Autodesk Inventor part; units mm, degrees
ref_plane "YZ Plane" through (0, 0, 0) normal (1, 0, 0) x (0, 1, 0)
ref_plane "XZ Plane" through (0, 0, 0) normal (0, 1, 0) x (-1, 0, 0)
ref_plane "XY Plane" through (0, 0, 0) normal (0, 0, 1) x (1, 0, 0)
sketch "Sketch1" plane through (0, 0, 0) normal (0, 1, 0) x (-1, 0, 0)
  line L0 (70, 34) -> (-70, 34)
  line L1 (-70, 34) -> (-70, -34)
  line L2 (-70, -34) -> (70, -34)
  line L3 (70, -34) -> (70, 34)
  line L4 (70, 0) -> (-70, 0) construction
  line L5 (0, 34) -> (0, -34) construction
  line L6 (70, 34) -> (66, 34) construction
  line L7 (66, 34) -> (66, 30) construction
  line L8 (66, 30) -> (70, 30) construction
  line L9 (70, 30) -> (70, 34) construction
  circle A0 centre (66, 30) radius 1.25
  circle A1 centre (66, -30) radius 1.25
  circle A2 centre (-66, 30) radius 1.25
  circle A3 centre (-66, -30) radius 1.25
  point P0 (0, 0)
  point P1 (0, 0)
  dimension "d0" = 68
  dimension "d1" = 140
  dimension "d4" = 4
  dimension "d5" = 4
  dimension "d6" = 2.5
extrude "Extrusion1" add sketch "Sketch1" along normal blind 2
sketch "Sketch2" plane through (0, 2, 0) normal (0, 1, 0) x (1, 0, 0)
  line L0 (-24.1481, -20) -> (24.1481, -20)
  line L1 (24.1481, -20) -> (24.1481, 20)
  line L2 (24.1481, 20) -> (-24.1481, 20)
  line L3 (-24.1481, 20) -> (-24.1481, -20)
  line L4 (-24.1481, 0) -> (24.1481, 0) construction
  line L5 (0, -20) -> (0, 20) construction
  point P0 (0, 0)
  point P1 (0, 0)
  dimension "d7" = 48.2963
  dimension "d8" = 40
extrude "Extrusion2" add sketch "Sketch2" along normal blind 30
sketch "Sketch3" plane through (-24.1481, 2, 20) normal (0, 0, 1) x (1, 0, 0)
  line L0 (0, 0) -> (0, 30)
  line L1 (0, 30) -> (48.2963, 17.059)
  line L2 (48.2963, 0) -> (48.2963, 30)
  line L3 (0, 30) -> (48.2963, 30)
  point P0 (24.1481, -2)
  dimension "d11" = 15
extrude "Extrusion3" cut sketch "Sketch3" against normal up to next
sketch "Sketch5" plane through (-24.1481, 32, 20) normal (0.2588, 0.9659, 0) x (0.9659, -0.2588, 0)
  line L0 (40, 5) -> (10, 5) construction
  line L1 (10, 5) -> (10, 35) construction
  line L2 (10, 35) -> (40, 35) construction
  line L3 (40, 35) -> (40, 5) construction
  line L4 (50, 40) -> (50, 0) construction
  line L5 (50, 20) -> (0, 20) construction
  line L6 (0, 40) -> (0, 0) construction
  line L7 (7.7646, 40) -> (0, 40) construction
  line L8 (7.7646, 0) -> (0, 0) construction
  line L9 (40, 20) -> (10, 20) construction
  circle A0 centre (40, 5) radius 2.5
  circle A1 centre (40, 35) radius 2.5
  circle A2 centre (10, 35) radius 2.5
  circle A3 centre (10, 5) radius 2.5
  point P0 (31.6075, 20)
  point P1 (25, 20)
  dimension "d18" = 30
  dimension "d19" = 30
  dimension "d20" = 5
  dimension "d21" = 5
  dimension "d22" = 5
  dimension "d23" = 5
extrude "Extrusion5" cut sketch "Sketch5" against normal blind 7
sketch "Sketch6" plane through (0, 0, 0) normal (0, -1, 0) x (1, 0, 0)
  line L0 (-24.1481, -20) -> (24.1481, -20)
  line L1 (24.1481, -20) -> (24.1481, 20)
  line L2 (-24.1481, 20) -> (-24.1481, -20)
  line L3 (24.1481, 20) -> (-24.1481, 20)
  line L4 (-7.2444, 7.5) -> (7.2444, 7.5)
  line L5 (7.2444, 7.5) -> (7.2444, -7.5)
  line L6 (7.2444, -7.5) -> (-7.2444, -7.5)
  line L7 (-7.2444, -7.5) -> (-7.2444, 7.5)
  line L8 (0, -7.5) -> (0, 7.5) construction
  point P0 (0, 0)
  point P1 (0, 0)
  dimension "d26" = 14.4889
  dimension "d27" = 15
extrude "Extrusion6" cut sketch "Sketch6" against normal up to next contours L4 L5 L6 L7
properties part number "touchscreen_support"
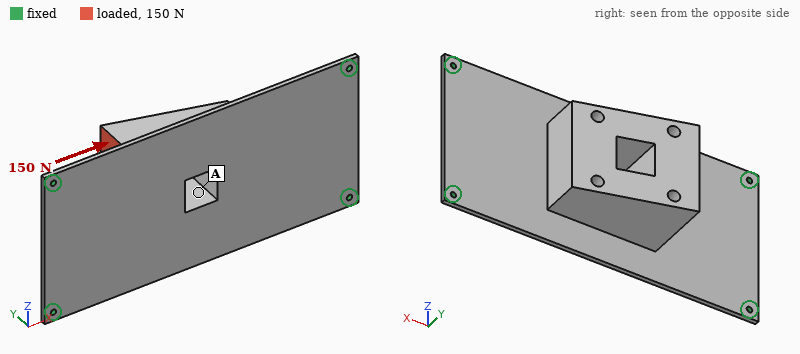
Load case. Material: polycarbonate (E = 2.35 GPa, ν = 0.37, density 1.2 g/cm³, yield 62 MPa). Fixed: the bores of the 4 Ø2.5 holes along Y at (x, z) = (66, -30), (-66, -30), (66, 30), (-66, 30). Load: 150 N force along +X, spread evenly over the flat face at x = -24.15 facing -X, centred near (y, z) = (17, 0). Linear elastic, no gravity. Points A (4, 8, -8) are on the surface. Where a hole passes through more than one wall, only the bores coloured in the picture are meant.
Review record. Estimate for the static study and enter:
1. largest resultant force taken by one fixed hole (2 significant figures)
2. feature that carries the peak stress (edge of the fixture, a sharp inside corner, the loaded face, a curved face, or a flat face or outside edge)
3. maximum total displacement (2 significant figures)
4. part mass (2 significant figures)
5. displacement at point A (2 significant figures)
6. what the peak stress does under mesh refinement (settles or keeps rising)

42 N
edge of the fixture
1.7 mm
70 g
0.37 mm
keeps rising
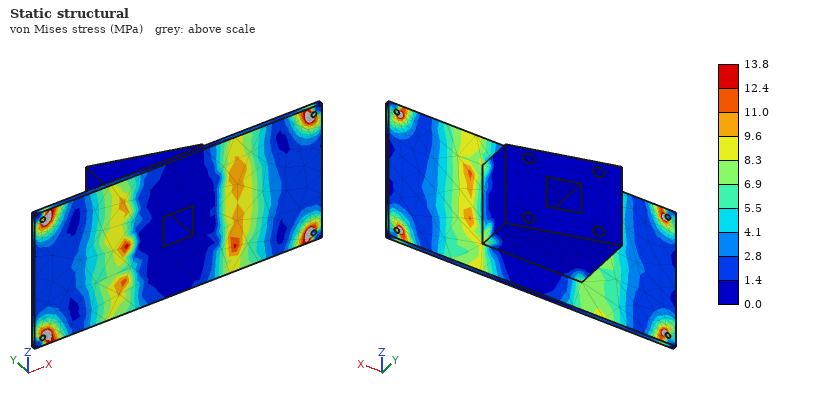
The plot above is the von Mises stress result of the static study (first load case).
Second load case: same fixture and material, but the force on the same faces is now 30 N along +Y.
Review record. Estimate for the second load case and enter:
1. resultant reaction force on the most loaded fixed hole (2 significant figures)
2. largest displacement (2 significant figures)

12 N
1.7 mm
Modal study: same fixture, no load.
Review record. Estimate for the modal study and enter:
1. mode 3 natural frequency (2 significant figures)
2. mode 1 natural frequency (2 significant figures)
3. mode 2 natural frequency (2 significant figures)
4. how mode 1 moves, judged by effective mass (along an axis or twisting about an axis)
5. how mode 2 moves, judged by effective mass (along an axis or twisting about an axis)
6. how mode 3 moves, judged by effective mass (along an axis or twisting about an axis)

230 Hz
95 Hz
140 Hz
along Y
along Z
along X
